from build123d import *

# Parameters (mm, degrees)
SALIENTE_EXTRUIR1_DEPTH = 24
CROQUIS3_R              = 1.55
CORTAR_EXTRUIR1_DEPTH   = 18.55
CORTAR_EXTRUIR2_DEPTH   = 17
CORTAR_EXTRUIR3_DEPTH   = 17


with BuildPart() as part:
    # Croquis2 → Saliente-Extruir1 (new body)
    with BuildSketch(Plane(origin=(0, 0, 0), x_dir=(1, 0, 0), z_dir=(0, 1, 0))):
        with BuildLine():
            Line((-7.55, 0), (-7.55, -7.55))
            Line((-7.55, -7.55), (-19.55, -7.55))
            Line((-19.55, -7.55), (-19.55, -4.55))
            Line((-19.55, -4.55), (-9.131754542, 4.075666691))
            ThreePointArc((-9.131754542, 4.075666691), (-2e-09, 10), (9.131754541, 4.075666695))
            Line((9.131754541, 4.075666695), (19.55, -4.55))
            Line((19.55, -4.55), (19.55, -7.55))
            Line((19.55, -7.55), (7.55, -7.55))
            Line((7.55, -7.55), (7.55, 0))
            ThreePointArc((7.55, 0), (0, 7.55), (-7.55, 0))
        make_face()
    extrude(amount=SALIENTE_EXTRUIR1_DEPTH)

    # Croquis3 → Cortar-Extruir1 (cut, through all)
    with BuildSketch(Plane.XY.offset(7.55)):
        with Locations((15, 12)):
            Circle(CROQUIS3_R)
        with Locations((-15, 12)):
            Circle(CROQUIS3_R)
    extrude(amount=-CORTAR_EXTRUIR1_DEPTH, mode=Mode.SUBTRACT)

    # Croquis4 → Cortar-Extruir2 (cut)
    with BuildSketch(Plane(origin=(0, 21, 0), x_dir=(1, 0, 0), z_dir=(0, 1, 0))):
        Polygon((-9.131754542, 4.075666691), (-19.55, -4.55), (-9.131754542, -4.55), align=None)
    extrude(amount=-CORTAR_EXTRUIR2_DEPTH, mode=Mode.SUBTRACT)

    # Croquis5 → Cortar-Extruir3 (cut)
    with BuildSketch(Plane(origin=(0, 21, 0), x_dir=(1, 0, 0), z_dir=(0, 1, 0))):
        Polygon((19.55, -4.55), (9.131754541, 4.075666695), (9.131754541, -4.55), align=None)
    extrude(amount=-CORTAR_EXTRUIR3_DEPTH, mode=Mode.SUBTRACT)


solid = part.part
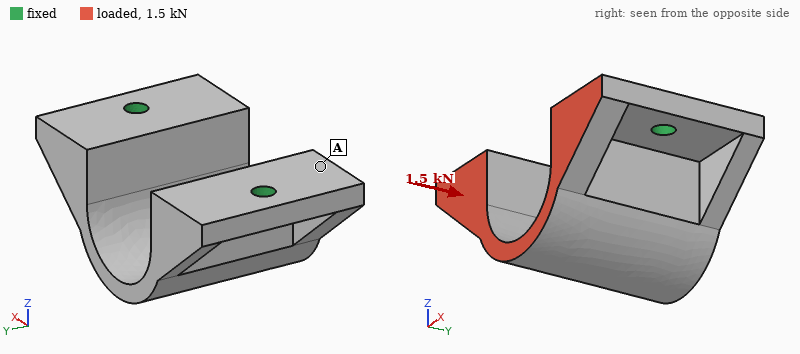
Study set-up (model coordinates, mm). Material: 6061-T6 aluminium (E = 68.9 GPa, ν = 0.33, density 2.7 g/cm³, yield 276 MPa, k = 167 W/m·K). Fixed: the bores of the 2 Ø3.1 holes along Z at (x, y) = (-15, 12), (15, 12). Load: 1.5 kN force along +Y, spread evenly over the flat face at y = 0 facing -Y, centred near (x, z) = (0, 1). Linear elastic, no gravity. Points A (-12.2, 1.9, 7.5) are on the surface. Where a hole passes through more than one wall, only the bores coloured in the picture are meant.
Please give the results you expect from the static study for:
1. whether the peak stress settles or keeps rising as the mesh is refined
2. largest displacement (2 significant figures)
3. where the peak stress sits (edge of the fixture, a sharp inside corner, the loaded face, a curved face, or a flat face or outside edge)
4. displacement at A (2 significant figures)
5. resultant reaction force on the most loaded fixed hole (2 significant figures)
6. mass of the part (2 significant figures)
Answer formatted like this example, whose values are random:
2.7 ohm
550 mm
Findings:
keeps rising
0.11 mm
edge of the fixture
0.045 mm
750 N
11 g
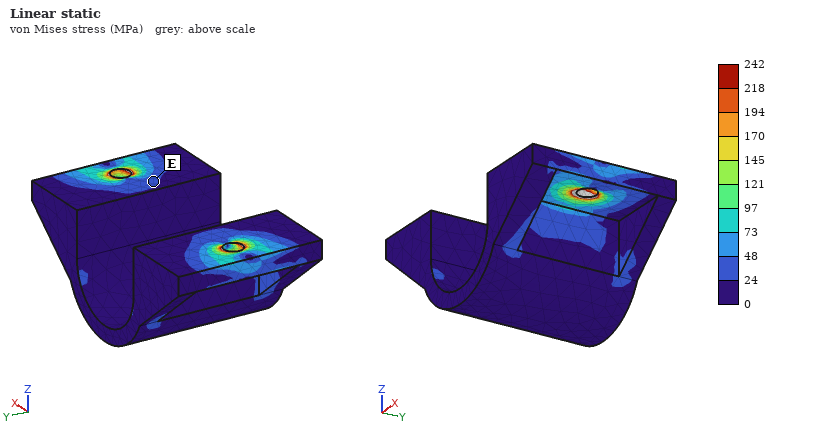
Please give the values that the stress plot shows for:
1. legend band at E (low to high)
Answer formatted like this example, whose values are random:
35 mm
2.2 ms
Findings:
24 to 48 MPa
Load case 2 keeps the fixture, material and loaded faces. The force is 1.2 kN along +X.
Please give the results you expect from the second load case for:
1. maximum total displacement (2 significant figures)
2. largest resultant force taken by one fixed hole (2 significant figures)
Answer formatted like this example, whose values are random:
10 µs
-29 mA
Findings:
70 µm
640 N
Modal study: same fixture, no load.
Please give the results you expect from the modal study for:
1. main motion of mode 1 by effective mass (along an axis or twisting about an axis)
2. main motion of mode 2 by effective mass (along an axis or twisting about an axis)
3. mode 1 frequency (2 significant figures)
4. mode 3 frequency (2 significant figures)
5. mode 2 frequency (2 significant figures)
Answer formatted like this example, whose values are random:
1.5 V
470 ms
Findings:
along Y
along X
5700 Hz
12 kHz
11 kHz
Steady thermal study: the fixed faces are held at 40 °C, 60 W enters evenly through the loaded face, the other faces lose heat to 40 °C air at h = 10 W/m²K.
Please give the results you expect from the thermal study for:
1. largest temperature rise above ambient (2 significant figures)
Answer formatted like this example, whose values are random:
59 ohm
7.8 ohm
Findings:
47 K
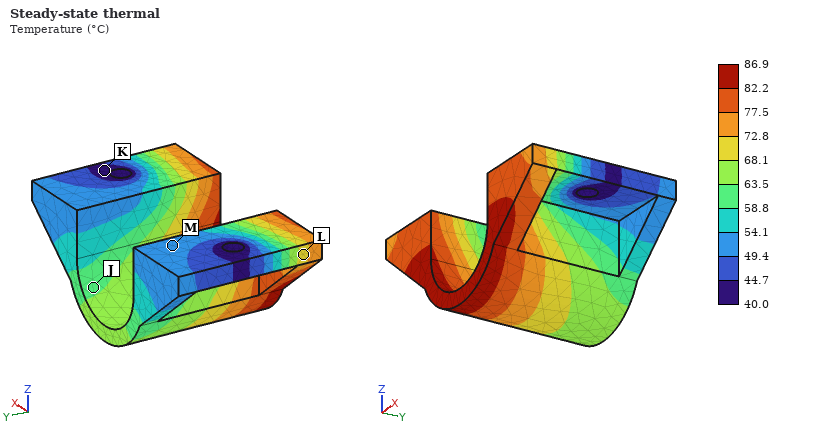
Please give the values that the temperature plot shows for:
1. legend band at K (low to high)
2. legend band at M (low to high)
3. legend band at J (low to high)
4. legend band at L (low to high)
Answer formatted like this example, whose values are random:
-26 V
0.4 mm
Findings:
40.0 to 44.7 °C
49.4 to 54.1 °C
58.8 to 63.5 °C
68.1 to 72.8 °C
